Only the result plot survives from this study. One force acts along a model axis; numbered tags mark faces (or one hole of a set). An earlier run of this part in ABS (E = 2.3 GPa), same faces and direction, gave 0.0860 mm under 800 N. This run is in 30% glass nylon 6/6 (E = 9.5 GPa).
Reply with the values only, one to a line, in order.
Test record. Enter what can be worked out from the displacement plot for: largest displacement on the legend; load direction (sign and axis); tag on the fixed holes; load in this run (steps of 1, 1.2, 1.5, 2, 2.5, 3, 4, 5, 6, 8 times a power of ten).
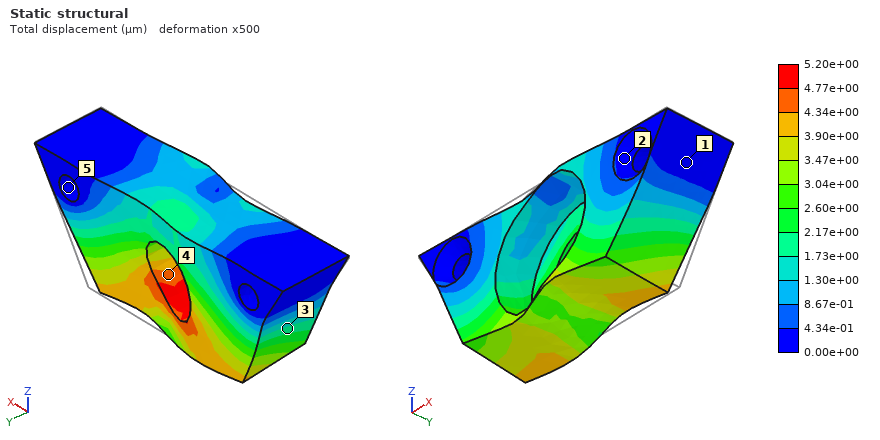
5.20e+00 µm
-X
5
200 N
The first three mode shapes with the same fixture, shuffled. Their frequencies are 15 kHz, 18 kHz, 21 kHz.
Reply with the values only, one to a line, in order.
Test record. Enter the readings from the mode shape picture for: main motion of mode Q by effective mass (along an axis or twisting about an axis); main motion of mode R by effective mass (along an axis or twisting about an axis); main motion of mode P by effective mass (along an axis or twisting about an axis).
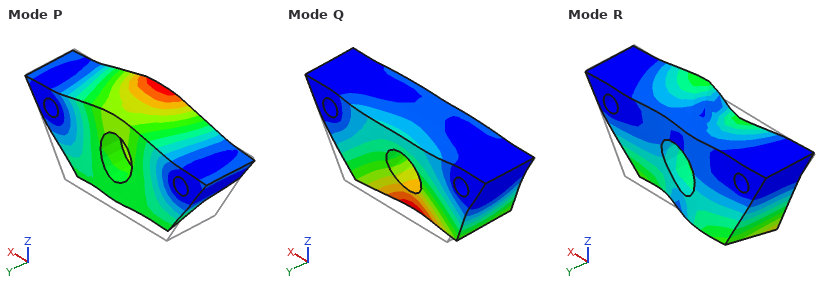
along Y
along X
along Z
